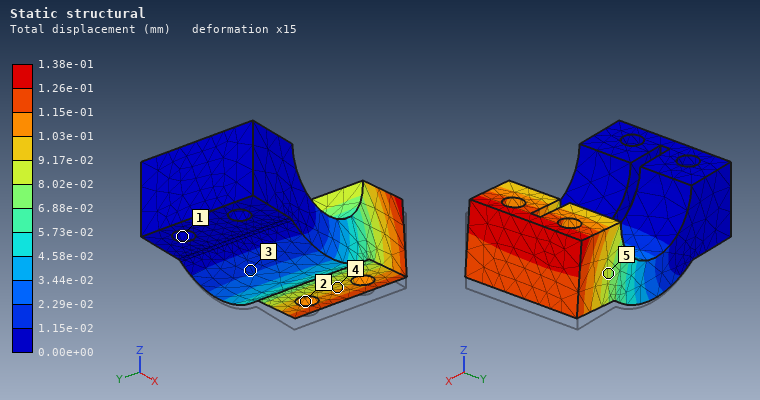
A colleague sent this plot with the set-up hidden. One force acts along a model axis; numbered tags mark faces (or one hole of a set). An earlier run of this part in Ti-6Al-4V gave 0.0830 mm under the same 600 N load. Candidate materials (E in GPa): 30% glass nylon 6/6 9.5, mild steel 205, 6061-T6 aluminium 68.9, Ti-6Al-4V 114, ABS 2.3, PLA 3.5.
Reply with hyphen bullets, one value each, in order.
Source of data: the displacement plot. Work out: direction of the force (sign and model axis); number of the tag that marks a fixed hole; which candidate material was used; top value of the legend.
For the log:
- +Z
- 1
- 6061-T6 aluminium
- 1.38e-01 mm
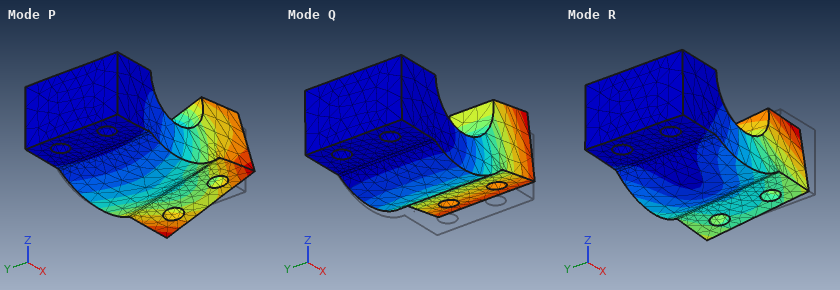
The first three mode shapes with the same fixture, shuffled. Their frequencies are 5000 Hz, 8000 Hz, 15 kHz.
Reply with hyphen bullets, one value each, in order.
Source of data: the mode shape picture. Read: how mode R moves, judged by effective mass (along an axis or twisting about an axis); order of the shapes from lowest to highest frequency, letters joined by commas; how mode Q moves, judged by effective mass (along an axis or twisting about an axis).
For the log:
- along Y
- Q, R, P
- along Z
